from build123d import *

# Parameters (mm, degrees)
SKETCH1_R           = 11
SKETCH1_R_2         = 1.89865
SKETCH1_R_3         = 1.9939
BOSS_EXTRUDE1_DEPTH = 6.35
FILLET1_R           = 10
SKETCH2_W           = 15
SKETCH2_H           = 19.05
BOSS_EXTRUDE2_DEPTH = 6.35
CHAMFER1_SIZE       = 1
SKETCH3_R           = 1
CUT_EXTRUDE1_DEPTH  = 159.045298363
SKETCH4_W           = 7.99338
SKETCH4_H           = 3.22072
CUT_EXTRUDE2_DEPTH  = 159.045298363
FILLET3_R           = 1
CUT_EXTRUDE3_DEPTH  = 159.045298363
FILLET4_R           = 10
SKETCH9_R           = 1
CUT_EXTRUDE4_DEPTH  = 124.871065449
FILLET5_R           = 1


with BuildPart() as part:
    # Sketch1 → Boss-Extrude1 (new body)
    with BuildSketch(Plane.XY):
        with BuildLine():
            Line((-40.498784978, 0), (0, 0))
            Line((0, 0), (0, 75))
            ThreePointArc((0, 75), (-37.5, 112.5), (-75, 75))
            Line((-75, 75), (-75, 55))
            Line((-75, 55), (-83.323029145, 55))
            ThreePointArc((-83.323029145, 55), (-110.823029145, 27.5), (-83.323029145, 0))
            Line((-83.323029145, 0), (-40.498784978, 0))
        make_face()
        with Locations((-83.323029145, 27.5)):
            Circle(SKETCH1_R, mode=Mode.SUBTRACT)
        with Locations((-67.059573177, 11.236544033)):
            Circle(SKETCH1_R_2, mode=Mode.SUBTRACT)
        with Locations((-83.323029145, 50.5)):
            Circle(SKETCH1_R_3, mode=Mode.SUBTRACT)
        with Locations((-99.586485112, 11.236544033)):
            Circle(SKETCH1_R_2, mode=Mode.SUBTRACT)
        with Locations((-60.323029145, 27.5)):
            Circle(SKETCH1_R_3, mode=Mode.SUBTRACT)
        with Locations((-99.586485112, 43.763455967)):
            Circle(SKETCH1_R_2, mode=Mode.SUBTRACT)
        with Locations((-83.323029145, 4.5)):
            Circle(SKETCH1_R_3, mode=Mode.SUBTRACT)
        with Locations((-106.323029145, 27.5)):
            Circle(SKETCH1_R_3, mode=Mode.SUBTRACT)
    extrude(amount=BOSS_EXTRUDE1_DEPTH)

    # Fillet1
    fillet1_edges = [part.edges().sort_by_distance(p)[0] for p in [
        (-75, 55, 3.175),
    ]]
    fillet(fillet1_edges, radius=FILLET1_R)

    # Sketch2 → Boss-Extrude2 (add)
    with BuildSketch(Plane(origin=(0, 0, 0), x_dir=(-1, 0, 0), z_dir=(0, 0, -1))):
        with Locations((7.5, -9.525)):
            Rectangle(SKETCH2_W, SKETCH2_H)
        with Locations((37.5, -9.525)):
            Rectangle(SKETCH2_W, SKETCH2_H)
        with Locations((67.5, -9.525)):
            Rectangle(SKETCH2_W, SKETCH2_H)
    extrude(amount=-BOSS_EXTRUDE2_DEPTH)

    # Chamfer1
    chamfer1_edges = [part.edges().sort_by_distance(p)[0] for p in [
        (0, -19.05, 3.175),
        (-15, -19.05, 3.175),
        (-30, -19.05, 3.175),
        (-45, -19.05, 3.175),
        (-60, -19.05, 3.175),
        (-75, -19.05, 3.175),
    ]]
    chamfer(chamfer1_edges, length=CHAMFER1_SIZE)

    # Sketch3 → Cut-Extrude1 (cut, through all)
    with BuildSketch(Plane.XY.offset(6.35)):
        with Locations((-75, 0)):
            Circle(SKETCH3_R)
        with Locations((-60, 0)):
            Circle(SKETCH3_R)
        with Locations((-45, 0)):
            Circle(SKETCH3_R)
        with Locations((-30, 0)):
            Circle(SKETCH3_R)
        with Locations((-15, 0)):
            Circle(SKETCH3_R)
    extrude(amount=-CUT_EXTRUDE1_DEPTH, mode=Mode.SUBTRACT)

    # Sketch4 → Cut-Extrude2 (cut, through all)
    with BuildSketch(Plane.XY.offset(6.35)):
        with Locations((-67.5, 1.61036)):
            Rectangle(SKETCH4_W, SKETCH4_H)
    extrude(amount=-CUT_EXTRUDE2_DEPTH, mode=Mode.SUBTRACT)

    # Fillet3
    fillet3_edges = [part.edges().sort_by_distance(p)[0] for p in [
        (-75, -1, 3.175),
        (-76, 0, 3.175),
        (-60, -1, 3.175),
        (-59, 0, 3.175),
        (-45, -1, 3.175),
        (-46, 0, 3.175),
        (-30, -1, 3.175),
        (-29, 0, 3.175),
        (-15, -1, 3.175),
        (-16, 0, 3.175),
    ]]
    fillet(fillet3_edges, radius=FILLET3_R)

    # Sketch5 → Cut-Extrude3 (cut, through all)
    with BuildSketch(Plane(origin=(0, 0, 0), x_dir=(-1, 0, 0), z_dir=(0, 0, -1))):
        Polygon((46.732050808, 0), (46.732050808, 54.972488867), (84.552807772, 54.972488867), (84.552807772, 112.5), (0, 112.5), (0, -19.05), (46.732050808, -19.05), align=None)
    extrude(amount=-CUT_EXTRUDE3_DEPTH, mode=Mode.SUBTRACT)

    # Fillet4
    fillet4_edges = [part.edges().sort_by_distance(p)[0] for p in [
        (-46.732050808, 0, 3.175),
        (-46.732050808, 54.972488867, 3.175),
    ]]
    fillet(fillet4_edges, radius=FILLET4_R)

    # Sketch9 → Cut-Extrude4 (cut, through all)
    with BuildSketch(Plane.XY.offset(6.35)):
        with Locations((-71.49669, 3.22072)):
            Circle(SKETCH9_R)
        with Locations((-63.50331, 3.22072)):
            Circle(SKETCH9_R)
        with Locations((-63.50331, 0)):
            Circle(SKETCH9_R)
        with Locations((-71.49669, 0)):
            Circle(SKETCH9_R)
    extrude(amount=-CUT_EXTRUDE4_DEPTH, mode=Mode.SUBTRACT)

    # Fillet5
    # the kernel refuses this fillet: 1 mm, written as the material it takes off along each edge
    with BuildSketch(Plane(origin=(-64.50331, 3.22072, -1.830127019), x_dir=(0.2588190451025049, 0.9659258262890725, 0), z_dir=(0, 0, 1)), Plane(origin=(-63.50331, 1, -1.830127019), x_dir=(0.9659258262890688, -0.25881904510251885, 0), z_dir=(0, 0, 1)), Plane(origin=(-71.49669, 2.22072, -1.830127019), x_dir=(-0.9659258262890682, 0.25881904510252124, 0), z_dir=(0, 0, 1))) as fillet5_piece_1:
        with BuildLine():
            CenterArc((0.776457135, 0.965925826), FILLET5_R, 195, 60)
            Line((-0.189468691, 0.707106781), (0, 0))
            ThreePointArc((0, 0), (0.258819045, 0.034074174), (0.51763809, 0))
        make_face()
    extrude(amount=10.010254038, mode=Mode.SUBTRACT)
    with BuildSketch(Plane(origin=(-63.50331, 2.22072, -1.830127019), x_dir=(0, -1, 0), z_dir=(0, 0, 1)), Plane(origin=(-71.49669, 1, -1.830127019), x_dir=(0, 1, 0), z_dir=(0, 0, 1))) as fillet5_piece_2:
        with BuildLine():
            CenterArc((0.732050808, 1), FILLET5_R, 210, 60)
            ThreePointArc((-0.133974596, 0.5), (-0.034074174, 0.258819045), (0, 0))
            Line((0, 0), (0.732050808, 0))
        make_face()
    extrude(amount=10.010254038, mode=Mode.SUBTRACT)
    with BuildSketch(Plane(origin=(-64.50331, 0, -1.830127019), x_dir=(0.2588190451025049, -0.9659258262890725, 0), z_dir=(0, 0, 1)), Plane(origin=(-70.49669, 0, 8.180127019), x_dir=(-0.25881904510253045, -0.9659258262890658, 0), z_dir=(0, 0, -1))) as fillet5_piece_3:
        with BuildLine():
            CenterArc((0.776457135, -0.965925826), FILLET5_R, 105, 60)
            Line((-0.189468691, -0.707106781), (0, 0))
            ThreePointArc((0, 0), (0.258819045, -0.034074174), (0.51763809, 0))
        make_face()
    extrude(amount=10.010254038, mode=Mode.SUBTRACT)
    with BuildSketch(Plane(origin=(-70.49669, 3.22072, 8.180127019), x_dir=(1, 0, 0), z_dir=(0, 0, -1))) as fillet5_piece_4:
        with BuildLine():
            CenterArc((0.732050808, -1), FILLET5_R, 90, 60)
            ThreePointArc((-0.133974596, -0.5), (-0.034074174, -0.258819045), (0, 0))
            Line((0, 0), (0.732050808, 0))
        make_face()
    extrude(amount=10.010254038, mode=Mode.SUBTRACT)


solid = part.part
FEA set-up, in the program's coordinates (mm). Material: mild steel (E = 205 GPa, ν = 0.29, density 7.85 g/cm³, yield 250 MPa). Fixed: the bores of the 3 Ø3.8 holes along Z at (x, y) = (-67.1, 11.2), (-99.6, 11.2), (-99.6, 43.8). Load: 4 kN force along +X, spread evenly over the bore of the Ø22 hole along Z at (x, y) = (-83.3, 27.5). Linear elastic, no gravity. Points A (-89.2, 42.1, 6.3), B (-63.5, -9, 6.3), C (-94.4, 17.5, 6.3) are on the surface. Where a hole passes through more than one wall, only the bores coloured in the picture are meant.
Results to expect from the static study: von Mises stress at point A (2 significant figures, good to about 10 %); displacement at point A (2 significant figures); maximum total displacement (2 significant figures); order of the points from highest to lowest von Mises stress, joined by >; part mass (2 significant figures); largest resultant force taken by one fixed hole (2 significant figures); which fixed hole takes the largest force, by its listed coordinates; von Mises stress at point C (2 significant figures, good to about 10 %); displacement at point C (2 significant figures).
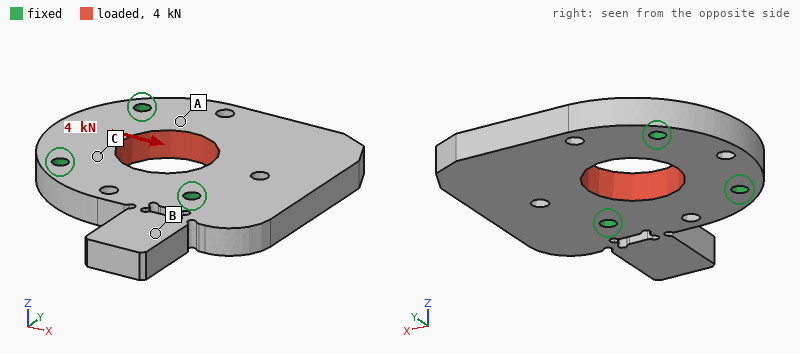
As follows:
19 MPa
1.0 µm
2.1 µm
A > C > B
150 g
1.8 kN
(-99.6, 43.8)
11 MPa
0.75 µm
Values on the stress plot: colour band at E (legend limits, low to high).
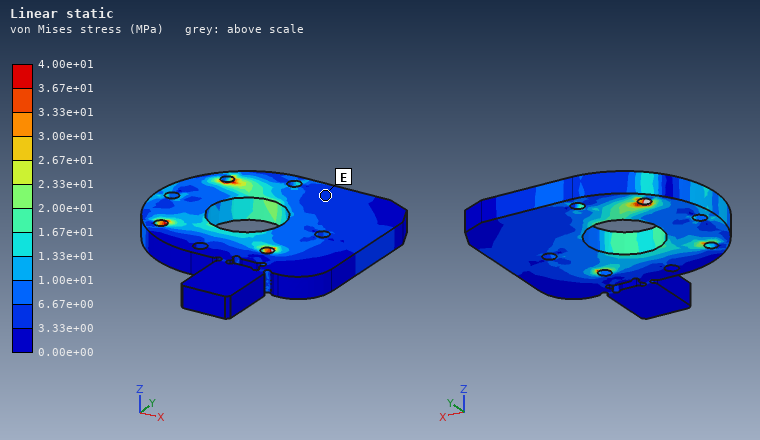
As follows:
3.33e+00 to 6.67e+00 MPa
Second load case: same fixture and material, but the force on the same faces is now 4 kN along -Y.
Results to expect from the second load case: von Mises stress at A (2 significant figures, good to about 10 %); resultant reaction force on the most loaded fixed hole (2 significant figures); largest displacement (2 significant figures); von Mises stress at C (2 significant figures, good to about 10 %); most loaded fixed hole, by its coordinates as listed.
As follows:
11 MPa
1.9 kN
2.4 µm
12 MPa
(-67.1, 11.2)
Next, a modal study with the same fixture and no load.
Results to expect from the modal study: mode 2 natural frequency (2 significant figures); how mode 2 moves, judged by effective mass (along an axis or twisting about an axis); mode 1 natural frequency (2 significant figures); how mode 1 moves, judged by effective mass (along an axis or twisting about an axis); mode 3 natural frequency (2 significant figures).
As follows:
4600 Hz
along Z
3500 Hz
along Z
9800 Hz
